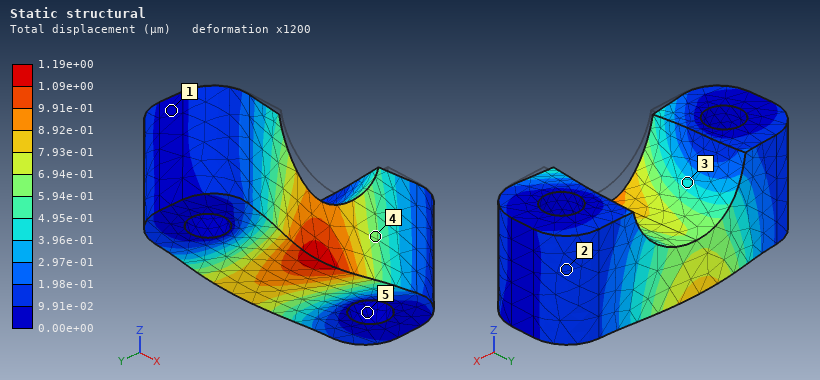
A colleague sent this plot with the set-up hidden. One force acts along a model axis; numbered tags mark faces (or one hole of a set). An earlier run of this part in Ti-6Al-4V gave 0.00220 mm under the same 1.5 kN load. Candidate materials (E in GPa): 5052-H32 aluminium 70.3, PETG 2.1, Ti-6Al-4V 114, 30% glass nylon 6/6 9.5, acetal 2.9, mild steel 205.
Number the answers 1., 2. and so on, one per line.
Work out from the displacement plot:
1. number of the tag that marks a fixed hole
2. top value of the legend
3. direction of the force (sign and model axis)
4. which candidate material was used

1. 5
2. 1.19e+00 µm
3. +Y
4. mild steel
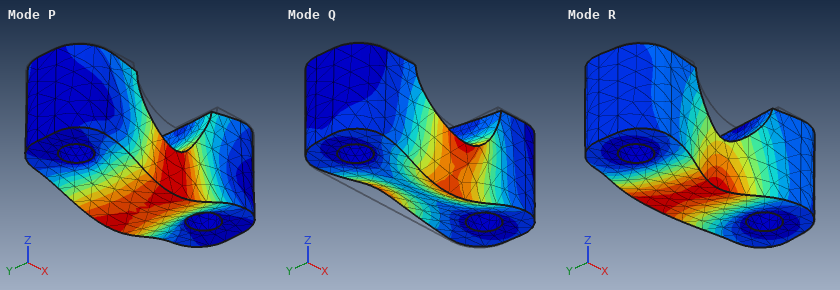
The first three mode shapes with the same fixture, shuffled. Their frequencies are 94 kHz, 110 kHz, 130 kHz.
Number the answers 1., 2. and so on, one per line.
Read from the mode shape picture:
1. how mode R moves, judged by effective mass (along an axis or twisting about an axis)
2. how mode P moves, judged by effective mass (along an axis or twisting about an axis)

1. along Y
2. along Z
